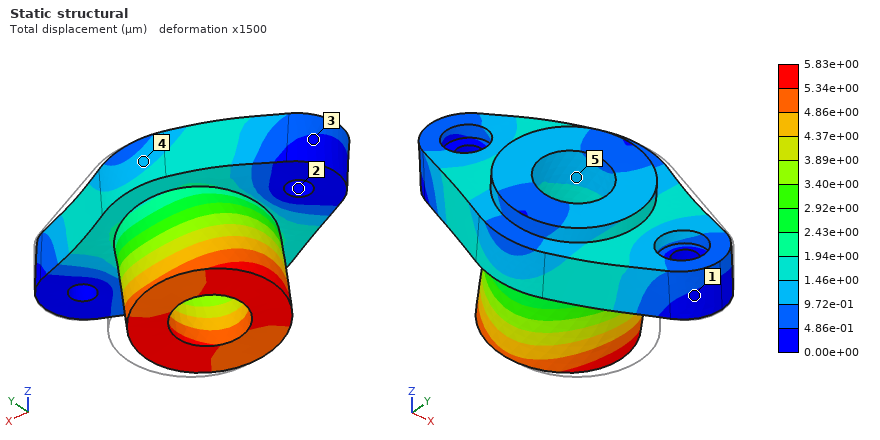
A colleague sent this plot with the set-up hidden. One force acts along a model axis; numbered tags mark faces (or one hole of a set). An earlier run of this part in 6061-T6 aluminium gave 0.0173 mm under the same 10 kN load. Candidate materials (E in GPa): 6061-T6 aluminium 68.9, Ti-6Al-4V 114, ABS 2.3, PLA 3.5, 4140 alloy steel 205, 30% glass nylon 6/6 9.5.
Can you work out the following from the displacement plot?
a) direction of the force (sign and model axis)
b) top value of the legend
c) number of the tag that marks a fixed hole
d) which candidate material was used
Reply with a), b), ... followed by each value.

a) -X
b) 5.83e+00 µm
c) 2
d) 4140 alloy steel
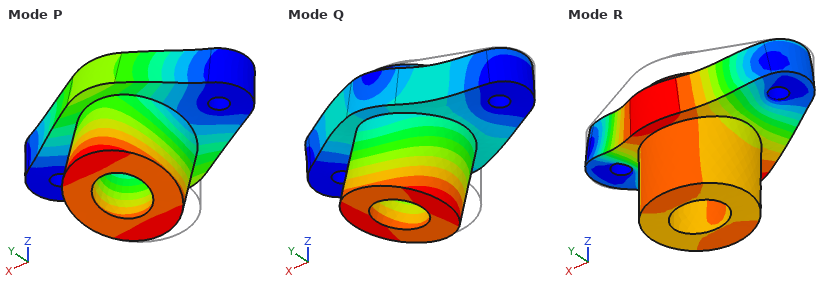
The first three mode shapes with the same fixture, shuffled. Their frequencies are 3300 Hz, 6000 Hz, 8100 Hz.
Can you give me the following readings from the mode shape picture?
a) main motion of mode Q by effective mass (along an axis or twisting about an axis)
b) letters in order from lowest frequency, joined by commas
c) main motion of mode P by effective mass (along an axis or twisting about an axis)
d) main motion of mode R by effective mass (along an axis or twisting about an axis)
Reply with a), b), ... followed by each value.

a) along X
b) P, R, Q
c) along Y
d) along Z
